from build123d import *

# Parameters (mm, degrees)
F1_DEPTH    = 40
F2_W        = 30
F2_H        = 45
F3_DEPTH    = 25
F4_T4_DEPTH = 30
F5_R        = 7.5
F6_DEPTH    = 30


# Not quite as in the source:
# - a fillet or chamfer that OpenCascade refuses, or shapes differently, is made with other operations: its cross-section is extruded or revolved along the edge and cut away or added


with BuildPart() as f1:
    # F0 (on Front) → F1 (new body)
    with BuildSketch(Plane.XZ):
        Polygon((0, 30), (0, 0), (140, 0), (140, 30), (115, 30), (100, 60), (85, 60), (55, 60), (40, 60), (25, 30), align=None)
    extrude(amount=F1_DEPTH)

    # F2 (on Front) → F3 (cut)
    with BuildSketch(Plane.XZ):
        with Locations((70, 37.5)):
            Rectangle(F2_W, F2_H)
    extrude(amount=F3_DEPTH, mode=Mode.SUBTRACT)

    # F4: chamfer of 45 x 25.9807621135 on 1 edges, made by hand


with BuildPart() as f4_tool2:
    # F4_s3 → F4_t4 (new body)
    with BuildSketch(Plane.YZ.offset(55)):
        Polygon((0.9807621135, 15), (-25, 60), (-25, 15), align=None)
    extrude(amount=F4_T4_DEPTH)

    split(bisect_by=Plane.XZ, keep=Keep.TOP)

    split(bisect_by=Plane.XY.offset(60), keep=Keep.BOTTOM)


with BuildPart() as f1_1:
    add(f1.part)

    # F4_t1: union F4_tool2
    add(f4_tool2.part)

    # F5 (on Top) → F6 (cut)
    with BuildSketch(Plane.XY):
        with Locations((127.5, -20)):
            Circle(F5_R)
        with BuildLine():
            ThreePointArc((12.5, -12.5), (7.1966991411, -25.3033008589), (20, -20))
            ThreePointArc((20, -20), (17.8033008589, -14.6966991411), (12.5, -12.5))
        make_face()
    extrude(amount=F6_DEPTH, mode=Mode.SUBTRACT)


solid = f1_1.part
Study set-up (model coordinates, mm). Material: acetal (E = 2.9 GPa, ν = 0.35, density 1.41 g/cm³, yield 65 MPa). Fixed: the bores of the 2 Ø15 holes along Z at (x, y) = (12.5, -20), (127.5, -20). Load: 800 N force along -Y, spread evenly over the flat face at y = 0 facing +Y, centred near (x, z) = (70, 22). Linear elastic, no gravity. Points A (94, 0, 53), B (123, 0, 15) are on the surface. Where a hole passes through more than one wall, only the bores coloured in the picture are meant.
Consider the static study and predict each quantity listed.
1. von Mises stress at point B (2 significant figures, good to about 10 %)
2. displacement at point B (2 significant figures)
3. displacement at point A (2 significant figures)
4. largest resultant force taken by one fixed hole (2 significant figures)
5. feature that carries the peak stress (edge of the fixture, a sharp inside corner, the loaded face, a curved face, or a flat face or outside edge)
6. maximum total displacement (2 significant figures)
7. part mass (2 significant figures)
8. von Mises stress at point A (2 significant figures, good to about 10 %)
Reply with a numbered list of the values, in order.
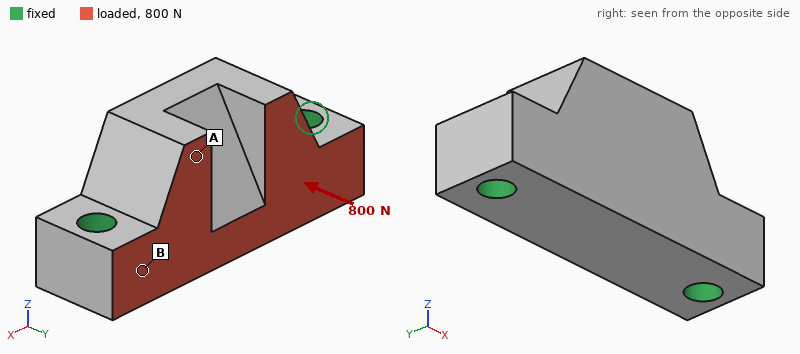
1. 0.57 MPa
2. 4.5 µm
3. 24 µm
4. 400 N
5. edge of the fixture
6. 28 µm
7. 330 g
8. 0.16 MPa
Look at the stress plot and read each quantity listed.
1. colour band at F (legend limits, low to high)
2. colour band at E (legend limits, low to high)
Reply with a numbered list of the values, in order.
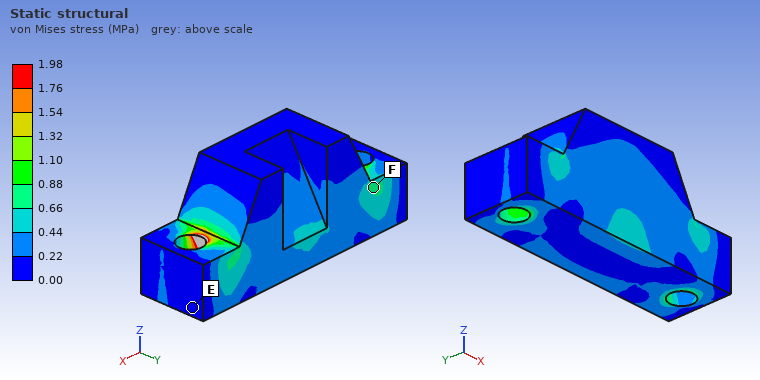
1. 0.66 to 0.88 MPa
2. 0.00 to 0.22 MPa
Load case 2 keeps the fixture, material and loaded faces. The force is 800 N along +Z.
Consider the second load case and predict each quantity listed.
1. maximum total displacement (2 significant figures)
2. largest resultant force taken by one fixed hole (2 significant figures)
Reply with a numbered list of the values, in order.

1. 37 µm
2. 410 N
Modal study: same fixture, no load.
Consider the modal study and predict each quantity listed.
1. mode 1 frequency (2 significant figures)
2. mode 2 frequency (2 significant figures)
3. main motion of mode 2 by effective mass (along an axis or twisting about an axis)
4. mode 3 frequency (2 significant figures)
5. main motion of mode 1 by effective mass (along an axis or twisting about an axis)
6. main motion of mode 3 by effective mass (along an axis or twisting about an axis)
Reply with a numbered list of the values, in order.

1. 1600 Hz
2. 2500 Hz
3. along Z
4. 2700 Hz
5. along Y
6. along Y
